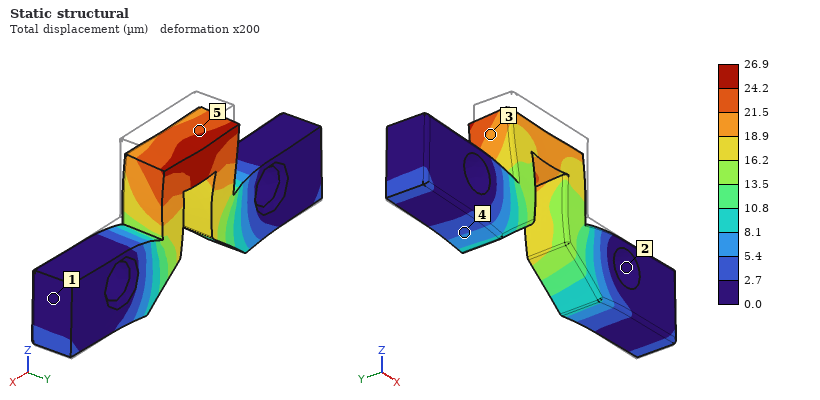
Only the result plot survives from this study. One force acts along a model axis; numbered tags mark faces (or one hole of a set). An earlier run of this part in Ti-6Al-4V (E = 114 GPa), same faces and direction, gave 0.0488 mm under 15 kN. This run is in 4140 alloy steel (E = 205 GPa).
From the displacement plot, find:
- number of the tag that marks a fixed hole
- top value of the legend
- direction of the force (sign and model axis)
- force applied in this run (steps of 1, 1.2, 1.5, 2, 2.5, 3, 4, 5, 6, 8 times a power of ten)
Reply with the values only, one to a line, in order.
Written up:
2
26.9 µm
-Z
15 kN
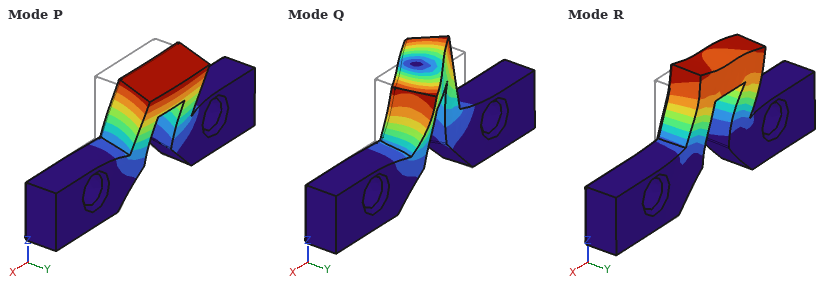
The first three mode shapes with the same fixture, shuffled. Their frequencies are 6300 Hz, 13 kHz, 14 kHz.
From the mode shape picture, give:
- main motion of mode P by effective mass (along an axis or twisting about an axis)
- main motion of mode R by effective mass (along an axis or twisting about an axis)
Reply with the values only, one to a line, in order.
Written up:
along Y
along X
